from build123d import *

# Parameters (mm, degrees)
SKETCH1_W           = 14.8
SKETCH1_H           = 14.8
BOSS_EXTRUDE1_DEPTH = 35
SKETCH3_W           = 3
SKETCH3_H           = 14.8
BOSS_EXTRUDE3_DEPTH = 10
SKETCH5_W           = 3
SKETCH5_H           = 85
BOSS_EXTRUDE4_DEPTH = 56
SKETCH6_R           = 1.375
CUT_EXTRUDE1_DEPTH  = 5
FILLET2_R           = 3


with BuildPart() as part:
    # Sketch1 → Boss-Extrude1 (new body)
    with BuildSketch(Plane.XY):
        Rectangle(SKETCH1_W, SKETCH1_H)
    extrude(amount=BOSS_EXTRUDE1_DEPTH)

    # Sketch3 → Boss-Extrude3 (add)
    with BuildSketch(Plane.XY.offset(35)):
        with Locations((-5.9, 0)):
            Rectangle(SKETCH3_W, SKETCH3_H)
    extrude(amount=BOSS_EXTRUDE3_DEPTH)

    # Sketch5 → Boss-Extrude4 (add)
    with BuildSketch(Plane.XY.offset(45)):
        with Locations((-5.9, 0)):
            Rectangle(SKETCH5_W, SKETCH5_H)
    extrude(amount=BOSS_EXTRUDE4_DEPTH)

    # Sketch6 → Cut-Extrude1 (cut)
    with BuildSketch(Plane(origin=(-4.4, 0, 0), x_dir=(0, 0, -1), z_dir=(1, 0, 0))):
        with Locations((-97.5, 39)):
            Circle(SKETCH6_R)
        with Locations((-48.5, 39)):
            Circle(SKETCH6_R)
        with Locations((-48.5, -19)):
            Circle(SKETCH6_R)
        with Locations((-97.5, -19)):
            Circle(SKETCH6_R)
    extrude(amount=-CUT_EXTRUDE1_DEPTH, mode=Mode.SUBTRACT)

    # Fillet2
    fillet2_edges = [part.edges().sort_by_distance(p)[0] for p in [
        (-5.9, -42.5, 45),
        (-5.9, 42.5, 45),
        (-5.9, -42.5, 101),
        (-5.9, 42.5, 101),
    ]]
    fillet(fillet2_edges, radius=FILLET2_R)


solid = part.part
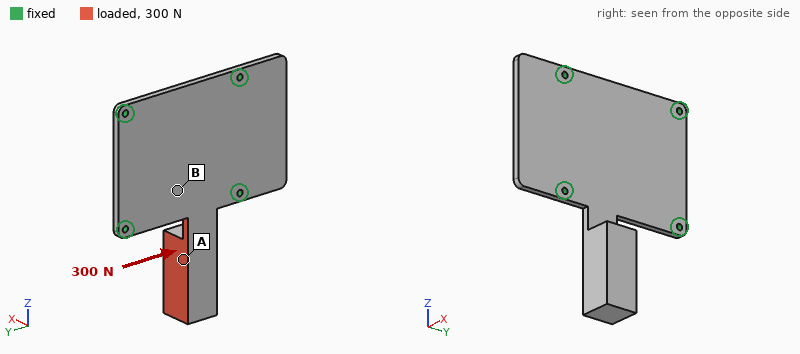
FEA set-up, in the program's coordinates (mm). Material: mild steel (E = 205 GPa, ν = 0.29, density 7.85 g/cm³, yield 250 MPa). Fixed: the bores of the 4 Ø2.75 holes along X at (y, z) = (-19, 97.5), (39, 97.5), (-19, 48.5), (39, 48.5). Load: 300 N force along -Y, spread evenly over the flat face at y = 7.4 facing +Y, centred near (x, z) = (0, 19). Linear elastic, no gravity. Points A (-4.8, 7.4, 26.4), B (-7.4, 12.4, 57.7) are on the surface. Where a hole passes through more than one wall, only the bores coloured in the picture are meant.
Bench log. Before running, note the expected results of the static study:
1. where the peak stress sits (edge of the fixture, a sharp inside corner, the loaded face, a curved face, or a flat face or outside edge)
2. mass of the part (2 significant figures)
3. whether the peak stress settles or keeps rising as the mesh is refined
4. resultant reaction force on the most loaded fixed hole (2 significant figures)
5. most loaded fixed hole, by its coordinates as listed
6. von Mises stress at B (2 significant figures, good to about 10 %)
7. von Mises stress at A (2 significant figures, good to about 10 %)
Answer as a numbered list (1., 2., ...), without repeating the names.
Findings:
1. a sharp inside corner
2. 180 g
3. keeps rising
4. 280 N
5. (-19, 48.5)
6. 19 MPa
7. 8.7 MPa
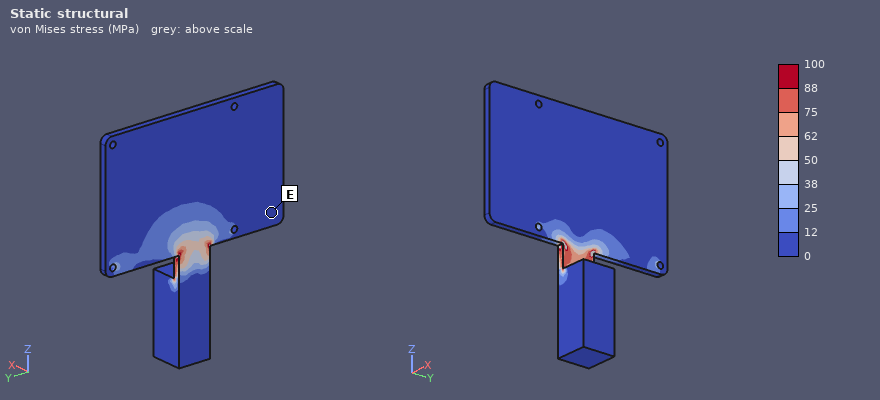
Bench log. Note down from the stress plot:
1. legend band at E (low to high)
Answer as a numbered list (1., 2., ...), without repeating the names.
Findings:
1. 0 to 12 MPa
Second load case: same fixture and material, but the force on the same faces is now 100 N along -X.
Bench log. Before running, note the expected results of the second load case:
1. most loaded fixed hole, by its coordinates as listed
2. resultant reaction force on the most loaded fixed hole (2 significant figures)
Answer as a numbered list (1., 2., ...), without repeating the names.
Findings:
1. (-19, 48.5)
2. 98 N
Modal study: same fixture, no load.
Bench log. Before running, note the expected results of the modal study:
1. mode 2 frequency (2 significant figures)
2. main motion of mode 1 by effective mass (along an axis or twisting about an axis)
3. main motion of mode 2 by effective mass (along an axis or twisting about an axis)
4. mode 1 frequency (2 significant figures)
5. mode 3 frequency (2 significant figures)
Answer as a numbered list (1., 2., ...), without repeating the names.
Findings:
1. 1600 Hz
2. along X
3. along Y
4. 410 Hz
5. 2800 Hz
